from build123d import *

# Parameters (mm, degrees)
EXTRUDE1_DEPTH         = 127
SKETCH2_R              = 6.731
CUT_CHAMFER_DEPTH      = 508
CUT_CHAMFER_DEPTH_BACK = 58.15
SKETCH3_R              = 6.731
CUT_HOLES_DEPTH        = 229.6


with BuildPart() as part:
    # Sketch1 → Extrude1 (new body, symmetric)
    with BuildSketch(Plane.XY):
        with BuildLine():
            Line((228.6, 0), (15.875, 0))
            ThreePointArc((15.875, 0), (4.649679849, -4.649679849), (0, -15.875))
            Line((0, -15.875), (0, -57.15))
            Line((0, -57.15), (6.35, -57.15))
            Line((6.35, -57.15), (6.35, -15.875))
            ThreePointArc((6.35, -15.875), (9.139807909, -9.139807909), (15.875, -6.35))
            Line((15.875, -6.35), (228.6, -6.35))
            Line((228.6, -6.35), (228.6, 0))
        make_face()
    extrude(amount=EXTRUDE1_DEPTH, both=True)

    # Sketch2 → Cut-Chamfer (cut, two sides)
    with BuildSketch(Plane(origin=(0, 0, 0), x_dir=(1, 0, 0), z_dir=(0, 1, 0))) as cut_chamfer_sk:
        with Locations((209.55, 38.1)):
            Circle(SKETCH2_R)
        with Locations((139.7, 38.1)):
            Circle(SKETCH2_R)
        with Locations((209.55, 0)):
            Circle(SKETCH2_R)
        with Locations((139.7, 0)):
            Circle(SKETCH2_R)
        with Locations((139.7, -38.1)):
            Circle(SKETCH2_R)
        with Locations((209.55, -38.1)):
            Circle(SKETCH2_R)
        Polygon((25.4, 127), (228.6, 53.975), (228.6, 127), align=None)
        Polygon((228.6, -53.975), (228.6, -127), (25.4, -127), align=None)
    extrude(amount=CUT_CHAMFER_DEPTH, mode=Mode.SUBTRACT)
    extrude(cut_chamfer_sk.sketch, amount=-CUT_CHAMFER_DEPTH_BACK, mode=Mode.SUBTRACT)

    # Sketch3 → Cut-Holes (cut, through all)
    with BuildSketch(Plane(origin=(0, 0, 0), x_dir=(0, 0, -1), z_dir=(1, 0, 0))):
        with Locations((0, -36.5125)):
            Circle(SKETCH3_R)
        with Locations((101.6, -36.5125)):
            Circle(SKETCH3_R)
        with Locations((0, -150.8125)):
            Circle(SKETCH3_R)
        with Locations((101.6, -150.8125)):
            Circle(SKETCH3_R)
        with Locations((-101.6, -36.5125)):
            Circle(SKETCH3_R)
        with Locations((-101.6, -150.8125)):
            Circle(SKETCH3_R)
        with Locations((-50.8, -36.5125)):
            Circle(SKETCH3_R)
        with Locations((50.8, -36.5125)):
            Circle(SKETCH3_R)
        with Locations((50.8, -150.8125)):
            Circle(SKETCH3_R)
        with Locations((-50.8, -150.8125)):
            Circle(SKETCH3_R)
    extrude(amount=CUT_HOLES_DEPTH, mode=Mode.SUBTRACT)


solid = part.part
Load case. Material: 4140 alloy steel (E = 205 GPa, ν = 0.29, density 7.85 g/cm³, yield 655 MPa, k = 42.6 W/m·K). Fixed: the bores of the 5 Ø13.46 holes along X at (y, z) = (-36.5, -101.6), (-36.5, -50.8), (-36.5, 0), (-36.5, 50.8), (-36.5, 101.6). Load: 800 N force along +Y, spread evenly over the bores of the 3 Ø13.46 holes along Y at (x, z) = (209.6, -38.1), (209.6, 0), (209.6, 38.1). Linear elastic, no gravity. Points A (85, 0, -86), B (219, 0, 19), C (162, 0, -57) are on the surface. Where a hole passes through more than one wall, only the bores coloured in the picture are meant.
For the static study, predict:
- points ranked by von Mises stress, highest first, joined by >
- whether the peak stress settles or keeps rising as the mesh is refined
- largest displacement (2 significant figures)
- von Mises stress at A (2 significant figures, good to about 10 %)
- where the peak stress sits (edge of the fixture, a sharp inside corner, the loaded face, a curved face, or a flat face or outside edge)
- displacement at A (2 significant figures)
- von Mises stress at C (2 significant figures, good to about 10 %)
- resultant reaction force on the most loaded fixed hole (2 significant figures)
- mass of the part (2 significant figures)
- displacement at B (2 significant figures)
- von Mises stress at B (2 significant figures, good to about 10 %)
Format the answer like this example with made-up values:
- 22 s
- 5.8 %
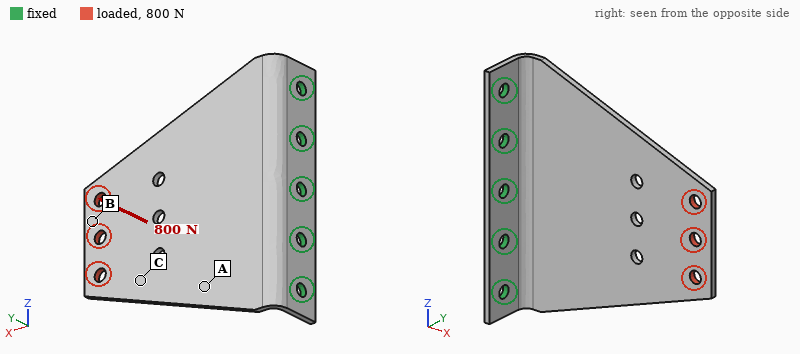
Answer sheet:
- A > C > B
- keeps rising
- 3.5 mm
- 74 MPa
- edge of the fixture
- 0.69 mm
- 44 MPa
- 410 N
- 2.7 kg
- 3.3 mm
- 16 MPa
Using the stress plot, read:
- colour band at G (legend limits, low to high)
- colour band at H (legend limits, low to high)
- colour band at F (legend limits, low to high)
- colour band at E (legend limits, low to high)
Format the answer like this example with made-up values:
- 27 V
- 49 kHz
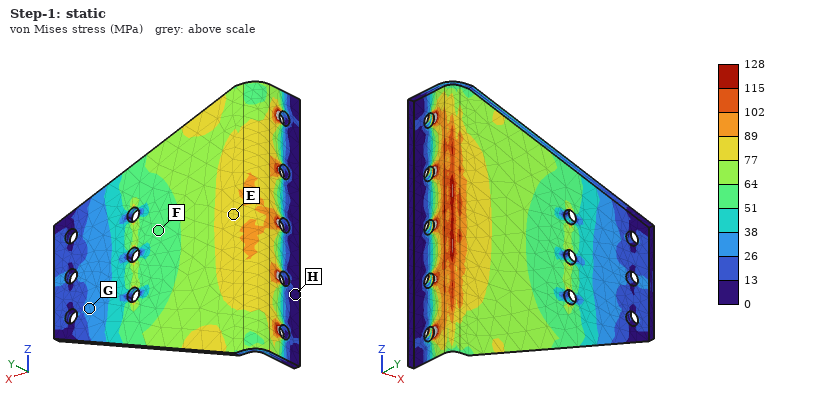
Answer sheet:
- 26 to 38 MPa
- 0 to 13 MPa
- 51 to 64 MPa
- 77 to 89 MPa
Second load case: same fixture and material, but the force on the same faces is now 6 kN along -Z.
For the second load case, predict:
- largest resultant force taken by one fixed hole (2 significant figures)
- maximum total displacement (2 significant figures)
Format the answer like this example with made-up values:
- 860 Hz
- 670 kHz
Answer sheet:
- 5.1 kN
- 0.43 mm
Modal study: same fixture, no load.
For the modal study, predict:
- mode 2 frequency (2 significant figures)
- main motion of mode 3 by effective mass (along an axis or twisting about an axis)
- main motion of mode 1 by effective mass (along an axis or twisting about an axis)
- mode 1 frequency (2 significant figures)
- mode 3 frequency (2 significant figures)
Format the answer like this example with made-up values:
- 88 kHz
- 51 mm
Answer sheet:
- 390 Hz
- along Y
- along Y
- 120 Hz
- 590 Hz
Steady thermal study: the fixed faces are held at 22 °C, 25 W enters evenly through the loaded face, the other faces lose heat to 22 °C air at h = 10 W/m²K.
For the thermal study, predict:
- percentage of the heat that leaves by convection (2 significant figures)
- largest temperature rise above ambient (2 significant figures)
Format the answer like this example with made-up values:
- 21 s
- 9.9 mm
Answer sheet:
- 74 %
- 67 K
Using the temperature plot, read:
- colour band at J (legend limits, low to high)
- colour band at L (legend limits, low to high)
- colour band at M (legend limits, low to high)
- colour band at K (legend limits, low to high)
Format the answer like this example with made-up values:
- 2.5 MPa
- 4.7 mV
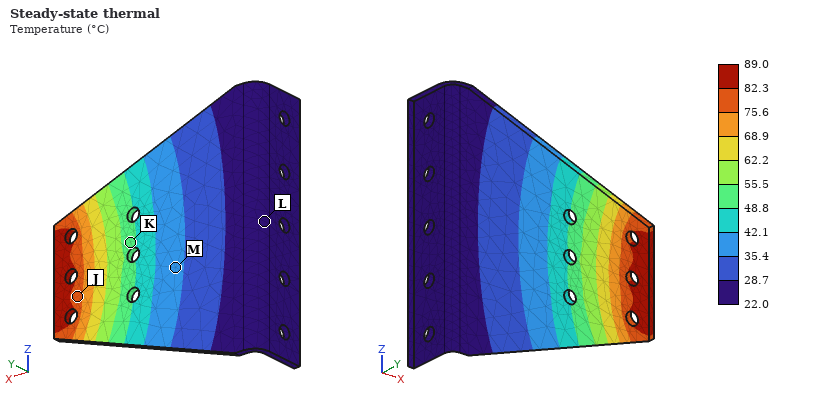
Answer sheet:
- 75.6 to 82.3 °C
- 22.0 to 28.7 °C
- 35.4 to 42.1 °C
- 48.8 to 55.5 °C
